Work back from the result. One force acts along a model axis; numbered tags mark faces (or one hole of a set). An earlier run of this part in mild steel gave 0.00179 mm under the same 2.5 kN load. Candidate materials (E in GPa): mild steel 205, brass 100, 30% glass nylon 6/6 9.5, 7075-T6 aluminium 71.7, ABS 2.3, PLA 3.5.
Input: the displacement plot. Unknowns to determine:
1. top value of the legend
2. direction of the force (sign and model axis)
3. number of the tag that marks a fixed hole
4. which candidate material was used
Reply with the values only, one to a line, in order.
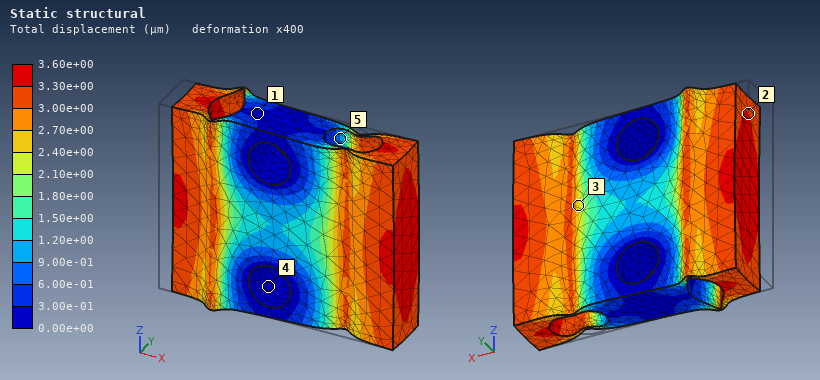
3.60e+00 µm
+X
4
brass
